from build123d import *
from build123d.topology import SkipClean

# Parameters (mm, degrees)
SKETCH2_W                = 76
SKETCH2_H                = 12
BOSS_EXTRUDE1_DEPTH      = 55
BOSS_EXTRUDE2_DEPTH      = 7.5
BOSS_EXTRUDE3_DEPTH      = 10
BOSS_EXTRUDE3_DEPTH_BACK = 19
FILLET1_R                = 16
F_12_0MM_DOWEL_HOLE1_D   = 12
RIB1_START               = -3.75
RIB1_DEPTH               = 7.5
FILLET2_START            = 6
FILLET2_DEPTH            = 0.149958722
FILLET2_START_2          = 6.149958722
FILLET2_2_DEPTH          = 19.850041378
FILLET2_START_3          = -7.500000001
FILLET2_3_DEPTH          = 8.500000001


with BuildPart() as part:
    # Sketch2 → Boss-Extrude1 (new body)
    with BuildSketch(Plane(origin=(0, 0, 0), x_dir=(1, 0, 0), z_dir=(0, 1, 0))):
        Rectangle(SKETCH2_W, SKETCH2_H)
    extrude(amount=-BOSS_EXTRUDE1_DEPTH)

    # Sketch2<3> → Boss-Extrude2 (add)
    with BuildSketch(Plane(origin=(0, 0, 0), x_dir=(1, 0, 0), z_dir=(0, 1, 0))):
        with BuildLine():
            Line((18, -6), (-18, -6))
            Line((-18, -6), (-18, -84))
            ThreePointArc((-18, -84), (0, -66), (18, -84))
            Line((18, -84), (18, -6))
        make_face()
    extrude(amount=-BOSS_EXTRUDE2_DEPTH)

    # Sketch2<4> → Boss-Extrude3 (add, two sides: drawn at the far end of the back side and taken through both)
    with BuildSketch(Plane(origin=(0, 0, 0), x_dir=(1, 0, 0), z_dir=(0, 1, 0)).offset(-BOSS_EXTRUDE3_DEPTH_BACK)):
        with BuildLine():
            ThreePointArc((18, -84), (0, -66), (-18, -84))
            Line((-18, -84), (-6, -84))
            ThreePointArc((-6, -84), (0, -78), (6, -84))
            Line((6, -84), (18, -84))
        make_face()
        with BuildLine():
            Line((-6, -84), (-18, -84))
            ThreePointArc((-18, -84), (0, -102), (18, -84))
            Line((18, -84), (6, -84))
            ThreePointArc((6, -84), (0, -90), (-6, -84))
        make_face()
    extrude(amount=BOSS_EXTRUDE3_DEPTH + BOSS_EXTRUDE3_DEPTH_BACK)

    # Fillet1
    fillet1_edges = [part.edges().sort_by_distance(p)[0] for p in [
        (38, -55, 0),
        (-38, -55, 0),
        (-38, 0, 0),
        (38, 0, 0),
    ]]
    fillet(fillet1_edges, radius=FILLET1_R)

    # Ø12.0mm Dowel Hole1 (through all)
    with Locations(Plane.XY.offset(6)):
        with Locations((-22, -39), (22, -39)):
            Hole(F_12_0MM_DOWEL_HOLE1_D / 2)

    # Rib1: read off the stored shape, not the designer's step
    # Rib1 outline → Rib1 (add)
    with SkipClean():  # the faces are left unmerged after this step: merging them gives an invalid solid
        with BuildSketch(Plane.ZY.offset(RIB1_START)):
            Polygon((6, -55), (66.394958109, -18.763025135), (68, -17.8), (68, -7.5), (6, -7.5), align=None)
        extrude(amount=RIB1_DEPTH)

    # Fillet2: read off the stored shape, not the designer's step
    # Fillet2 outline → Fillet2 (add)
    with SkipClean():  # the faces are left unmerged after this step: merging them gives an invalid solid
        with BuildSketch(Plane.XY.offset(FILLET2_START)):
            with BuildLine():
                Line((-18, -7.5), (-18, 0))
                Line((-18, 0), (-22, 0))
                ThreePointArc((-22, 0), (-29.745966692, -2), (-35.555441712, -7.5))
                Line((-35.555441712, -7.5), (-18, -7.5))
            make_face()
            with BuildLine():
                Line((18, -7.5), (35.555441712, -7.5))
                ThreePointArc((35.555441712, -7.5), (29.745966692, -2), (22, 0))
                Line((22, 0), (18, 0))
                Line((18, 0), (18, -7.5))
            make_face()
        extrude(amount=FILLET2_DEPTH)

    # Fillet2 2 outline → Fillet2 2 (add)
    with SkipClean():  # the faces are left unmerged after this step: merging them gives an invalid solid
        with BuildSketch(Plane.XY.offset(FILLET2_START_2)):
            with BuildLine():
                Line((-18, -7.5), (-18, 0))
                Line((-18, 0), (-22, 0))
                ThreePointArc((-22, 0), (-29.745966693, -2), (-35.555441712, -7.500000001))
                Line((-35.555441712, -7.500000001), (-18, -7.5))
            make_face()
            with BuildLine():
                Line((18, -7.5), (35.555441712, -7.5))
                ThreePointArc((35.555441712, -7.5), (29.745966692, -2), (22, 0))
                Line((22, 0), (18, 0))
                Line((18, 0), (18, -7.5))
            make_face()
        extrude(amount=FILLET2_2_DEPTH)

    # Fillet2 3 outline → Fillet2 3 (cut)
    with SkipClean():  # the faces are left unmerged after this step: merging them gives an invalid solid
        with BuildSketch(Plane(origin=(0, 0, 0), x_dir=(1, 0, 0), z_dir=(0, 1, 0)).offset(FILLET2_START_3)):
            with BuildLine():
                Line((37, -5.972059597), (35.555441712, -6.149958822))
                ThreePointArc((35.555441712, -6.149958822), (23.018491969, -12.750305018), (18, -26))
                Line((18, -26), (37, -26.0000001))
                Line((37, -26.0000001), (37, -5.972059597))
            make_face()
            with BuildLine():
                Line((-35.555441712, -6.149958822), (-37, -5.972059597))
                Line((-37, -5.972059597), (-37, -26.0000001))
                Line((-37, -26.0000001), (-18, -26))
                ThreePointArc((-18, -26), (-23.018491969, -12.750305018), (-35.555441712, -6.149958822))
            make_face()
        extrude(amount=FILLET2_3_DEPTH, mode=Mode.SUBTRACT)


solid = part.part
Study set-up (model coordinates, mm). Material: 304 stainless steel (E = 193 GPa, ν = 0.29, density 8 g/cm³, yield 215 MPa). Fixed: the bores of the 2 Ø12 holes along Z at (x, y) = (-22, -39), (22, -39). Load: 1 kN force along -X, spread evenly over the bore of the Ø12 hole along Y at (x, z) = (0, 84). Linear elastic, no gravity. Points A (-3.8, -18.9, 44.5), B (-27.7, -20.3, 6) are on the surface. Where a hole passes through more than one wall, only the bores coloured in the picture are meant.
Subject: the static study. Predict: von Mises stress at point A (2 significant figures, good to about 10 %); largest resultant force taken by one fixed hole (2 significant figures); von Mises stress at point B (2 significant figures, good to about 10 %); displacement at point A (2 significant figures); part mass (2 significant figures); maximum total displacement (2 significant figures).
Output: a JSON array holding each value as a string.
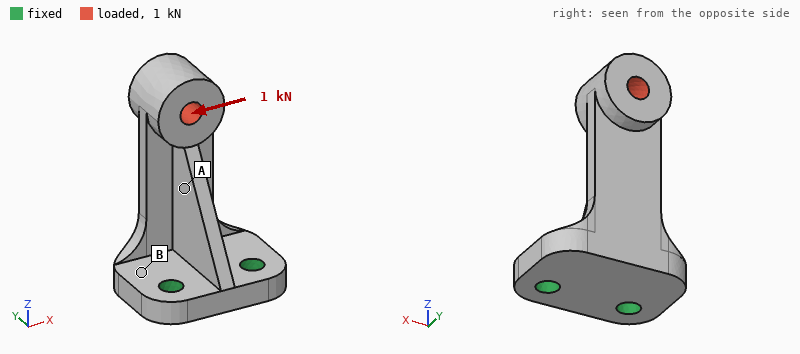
["8.0 MPa", "1.9 kN", "17 MPa", "25 µm", "820 g", "78 µm"]
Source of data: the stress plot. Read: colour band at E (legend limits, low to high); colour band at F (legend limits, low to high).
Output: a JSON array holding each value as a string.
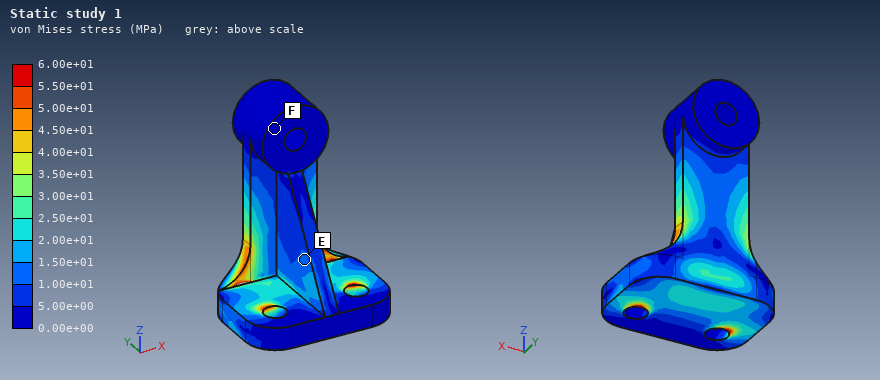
["1.00e+01 to 1.50e+01 MPa", "0.00e+00 to 5.00e+00 MPa"]
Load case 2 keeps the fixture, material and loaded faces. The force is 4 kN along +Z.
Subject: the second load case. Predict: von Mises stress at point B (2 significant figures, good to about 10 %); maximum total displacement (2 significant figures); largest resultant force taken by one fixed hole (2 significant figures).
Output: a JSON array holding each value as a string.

["23 MPa", "73 µm", "2.0 kN"]
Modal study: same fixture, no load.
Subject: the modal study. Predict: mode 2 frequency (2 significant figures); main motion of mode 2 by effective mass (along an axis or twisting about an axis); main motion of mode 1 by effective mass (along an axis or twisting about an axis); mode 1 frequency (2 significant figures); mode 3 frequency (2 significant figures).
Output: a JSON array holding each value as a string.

["1400 Hz", "along Y", "along X", "1300 Hz", "2800 Hz"]
